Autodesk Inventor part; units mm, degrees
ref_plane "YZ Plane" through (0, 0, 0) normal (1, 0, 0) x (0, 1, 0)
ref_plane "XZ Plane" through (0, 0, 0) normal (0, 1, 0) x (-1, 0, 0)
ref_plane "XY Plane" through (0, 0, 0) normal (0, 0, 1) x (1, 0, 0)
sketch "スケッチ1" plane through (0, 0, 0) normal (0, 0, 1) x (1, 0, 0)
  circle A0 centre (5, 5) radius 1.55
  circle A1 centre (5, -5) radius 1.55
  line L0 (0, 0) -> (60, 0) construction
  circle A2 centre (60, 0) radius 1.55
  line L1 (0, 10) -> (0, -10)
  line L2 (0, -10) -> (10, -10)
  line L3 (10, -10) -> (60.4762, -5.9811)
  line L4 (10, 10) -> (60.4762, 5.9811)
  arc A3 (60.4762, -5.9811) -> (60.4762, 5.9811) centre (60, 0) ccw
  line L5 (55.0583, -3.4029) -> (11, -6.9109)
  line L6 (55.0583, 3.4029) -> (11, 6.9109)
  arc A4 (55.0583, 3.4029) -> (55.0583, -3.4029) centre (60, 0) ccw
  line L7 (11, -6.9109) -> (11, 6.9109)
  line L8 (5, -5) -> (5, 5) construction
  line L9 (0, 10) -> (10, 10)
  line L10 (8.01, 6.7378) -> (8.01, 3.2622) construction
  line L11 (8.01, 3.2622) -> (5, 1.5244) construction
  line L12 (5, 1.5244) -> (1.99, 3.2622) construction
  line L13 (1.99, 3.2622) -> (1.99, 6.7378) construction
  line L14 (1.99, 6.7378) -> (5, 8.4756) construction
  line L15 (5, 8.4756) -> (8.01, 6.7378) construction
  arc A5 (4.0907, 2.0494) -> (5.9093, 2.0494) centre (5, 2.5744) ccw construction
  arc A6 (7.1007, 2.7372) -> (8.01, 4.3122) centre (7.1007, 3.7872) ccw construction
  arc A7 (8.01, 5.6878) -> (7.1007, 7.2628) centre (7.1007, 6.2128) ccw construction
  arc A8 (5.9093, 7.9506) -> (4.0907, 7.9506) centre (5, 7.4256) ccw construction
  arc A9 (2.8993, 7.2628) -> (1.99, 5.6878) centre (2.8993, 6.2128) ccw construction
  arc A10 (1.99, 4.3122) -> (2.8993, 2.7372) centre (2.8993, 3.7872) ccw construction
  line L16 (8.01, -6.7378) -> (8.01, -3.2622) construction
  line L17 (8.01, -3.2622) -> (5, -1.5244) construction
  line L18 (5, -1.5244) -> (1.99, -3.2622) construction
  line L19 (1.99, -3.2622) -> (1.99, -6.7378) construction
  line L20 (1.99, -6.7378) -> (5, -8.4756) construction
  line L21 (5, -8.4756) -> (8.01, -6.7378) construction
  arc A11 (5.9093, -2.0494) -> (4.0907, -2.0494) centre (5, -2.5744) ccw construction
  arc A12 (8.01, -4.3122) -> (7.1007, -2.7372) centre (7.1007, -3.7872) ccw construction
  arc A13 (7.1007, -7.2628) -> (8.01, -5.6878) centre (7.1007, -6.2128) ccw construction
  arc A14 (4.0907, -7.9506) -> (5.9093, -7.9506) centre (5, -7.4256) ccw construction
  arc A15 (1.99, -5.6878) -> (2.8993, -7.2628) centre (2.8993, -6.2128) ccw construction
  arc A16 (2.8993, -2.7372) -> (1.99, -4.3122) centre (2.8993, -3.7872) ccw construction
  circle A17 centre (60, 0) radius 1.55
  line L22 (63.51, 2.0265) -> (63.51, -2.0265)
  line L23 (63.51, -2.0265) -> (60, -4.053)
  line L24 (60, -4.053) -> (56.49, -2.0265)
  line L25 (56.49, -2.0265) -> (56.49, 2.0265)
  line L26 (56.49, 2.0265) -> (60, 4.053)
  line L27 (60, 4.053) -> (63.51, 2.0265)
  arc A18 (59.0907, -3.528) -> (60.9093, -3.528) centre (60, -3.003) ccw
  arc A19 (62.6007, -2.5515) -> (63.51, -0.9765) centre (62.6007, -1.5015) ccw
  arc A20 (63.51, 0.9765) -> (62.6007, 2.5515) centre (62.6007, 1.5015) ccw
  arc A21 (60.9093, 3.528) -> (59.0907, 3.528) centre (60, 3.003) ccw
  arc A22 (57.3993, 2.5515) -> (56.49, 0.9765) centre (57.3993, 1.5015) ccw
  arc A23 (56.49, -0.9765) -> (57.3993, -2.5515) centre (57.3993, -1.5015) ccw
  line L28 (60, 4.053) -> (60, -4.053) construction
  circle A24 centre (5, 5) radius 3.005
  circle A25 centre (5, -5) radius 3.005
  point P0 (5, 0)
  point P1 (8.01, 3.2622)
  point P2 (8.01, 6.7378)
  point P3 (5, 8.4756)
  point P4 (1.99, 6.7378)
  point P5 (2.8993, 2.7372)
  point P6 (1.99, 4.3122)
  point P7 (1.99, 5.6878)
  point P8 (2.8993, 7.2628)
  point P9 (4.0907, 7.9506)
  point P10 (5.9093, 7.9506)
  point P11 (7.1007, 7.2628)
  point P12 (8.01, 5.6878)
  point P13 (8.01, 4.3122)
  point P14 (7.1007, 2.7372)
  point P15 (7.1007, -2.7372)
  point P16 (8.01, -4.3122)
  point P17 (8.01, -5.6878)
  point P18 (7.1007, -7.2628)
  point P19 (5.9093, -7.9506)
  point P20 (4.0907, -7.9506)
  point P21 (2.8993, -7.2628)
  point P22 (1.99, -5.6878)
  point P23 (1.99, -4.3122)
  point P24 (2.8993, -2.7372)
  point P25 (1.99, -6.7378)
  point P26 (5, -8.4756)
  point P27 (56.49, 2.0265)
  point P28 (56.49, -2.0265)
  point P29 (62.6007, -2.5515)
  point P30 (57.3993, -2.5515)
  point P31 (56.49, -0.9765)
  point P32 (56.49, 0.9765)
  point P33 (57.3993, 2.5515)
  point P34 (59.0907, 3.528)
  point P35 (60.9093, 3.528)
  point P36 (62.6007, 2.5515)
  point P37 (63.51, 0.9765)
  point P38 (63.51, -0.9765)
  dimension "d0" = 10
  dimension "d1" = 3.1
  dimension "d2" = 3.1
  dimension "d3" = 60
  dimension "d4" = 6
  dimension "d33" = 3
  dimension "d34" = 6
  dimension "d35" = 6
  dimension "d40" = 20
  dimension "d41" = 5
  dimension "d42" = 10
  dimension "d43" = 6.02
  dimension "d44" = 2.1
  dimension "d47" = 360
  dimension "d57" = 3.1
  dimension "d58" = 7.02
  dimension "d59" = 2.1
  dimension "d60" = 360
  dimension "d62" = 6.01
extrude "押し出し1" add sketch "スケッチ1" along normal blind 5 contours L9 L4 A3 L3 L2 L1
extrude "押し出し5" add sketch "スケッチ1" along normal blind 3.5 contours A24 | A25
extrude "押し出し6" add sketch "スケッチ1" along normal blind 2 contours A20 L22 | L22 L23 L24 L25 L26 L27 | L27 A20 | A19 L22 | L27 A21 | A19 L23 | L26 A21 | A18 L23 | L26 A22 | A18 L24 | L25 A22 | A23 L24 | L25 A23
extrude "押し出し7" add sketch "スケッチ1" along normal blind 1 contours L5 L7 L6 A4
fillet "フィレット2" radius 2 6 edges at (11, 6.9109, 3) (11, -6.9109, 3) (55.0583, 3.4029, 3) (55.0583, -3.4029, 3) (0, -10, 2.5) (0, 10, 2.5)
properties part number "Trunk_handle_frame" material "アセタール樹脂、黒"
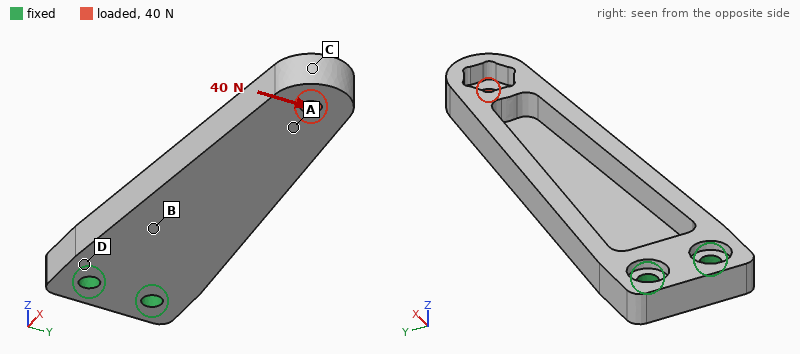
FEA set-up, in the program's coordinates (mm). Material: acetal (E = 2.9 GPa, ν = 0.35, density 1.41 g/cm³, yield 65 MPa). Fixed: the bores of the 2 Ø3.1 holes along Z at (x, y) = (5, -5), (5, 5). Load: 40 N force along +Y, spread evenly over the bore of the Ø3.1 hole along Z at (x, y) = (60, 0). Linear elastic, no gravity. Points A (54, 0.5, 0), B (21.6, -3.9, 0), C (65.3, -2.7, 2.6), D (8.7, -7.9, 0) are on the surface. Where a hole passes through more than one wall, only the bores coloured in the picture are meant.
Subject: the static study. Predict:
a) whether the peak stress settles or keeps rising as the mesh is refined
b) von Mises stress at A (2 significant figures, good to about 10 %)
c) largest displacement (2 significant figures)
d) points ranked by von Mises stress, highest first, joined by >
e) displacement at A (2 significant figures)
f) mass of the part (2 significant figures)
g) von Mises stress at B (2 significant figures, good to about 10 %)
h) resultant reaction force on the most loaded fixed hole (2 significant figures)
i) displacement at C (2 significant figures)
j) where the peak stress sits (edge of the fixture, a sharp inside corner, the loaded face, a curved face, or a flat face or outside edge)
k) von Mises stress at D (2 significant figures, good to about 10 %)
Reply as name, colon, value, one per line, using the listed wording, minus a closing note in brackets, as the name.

whether the peak stress settles or keeps rising as the mesh is refined: keeps rising
von Mises stress at A: 3.1 MPa
largest displacement: 0.66 mm
points ranked by von Mises stress, highest first, joined by >: D > B > A > C
displacement at A: 0.44 mm
mass of the part: 4.5 g
von Mises stress at B: 4.4 MPa
resultant reaction force on the most loaded fixed hole: 180 N
displacement at C: 0.62 mm
where the peak stress sits: edge of the fixture
von Mises stress at D: 6.7 MPa
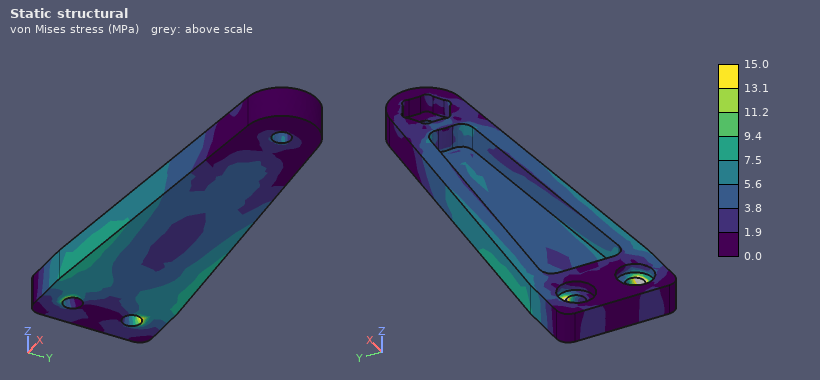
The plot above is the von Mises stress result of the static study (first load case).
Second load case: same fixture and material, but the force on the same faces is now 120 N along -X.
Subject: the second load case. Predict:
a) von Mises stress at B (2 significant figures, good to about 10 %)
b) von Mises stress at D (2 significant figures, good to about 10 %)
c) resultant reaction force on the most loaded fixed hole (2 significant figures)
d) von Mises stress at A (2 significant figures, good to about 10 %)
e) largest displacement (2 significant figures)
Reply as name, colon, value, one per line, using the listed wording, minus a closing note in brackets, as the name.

von Mises stress at B: 5.2 MPa
von Mises stress at D: 3.6 MPa
resultant reaction force on the most loaded fixed hole: 60 N
von Mises stress at A: 7.3 MPa
largest displacement: 0.72 mm
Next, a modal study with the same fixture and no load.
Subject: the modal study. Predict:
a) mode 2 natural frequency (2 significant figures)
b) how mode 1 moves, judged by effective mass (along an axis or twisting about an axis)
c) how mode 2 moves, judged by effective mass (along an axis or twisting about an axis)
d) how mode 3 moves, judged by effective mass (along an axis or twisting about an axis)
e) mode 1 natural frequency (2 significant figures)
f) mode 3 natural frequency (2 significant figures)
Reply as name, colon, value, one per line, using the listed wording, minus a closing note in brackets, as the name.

mode 2 natural frequency: 1000 Hz
how mode 1 moves, judged by effective mass: along Z
how mode 2 moves, judged by effective mass: along Y
how mode 3 moves, judged by effective mass: along Y
mode 1 natural frequency: 340 Hz
mode 3 natural frequency: 1600 Hz
